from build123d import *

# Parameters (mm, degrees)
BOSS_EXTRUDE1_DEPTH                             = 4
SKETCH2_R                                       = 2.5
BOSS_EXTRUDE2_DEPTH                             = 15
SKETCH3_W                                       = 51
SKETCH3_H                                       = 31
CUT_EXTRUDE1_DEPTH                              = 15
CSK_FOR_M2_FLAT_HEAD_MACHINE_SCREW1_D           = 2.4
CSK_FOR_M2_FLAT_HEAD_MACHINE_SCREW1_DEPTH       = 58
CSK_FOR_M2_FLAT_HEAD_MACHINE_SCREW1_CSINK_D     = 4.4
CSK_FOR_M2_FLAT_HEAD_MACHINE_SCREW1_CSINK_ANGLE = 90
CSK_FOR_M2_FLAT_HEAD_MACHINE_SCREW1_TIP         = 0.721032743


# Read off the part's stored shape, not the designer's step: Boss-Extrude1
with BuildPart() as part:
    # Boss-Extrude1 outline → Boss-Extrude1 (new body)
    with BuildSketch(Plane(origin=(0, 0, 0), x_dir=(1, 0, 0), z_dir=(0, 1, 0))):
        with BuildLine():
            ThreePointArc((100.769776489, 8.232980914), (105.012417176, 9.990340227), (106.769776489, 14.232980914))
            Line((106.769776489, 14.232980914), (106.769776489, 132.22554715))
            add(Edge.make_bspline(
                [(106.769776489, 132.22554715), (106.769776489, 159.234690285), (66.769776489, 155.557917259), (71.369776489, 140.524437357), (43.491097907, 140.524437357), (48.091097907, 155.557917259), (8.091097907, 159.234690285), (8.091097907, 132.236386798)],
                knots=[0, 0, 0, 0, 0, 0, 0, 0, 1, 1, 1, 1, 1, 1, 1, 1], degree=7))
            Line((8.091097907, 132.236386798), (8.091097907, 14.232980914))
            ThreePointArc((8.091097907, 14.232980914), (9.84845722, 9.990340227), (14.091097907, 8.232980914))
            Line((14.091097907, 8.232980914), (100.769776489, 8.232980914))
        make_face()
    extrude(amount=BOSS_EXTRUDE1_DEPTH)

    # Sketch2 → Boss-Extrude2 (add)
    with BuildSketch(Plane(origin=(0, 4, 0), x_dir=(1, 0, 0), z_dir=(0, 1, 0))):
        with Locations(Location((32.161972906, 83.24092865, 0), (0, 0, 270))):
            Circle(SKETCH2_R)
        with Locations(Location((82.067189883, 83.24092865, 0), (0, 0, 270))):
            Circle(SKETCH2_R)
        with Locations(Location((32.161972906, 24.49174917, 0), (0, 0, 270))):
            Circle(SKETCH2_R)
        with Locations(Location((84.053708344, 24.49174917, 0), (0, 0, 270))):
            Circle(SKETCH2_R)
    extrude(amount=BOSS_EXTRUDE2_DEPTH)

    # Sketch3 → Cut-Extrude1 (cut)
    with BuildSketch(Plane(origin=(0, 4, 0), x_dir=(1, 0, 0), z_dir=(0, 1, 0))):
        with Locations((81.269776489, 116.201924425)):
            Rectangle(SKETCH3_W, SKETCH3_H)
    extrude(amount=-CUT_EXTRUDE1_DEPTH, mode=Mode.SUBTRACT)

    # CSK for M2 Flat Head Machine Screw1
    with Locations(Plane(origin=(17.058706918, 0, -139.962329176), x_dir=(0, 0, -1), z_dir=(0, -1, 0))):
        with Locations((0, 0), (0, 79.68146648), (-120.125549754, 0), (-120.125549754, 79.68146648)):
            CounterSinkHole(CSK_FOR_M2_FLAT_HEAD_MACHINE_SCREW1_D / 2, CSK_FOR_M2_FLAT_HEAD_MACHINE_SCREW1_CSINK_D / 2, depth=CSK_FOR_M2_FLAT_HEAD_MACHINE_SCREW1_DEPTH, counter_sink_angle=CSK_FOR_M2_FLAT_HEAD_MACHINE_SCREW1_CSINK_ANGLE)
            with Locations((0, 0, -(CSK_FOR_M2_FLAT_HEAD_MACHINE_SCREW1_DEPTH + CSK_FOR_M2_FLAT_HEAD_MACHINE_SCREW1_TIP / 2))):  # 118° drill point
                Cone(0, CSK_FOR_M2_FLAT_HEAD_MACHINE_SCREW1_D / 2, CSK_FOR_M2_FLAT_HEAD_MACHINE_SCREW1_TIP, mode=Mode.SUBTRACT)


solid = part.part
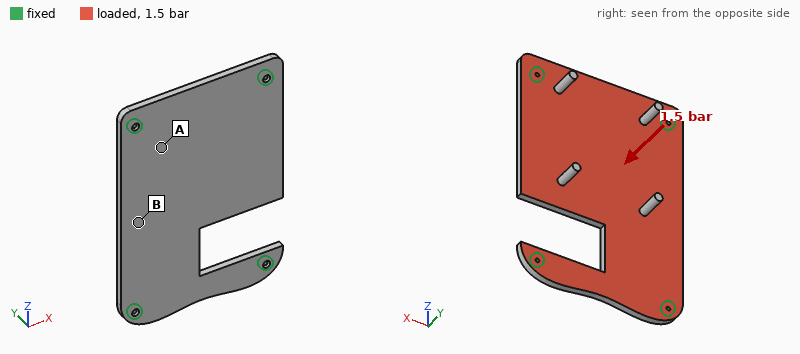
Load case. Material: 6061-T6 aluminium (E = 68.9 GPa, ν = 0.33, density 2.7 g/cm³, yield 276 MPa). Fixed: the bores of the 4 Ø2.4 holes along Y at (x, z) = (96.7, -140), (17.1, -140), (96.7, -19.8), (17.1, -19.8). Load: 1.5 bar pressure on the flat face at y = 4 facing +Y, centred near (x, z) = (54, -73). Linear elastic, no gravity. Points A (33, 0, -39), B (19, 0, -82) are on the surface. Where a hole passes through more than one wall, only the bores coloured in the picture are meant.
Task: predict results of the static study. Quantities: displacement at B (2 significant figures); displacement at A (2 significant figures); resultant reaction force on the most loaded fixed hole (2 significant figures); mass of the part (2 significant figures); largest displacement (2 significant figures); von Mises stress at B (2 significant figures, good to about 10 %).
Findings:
0.43 mm
0.22 mm
650 N
130 g
1.2 mm
53 MPa
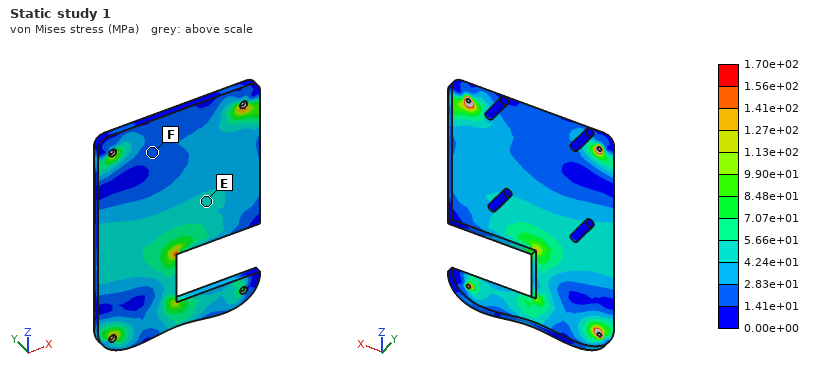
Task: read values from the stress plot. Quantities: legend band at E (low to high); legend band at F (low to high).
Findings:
4.24e+01 to 5.66e+01 MPa
1.41e+01 to 2.83e+01 MPa
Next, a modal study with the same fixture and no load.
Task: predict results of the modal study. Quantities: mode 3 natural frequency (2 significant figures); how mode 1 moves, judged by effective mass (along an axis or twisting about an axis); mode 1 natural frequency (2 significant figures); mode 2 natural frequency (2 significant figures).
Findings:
2400 Hz
along Y
760 Hz
1400 Hz
